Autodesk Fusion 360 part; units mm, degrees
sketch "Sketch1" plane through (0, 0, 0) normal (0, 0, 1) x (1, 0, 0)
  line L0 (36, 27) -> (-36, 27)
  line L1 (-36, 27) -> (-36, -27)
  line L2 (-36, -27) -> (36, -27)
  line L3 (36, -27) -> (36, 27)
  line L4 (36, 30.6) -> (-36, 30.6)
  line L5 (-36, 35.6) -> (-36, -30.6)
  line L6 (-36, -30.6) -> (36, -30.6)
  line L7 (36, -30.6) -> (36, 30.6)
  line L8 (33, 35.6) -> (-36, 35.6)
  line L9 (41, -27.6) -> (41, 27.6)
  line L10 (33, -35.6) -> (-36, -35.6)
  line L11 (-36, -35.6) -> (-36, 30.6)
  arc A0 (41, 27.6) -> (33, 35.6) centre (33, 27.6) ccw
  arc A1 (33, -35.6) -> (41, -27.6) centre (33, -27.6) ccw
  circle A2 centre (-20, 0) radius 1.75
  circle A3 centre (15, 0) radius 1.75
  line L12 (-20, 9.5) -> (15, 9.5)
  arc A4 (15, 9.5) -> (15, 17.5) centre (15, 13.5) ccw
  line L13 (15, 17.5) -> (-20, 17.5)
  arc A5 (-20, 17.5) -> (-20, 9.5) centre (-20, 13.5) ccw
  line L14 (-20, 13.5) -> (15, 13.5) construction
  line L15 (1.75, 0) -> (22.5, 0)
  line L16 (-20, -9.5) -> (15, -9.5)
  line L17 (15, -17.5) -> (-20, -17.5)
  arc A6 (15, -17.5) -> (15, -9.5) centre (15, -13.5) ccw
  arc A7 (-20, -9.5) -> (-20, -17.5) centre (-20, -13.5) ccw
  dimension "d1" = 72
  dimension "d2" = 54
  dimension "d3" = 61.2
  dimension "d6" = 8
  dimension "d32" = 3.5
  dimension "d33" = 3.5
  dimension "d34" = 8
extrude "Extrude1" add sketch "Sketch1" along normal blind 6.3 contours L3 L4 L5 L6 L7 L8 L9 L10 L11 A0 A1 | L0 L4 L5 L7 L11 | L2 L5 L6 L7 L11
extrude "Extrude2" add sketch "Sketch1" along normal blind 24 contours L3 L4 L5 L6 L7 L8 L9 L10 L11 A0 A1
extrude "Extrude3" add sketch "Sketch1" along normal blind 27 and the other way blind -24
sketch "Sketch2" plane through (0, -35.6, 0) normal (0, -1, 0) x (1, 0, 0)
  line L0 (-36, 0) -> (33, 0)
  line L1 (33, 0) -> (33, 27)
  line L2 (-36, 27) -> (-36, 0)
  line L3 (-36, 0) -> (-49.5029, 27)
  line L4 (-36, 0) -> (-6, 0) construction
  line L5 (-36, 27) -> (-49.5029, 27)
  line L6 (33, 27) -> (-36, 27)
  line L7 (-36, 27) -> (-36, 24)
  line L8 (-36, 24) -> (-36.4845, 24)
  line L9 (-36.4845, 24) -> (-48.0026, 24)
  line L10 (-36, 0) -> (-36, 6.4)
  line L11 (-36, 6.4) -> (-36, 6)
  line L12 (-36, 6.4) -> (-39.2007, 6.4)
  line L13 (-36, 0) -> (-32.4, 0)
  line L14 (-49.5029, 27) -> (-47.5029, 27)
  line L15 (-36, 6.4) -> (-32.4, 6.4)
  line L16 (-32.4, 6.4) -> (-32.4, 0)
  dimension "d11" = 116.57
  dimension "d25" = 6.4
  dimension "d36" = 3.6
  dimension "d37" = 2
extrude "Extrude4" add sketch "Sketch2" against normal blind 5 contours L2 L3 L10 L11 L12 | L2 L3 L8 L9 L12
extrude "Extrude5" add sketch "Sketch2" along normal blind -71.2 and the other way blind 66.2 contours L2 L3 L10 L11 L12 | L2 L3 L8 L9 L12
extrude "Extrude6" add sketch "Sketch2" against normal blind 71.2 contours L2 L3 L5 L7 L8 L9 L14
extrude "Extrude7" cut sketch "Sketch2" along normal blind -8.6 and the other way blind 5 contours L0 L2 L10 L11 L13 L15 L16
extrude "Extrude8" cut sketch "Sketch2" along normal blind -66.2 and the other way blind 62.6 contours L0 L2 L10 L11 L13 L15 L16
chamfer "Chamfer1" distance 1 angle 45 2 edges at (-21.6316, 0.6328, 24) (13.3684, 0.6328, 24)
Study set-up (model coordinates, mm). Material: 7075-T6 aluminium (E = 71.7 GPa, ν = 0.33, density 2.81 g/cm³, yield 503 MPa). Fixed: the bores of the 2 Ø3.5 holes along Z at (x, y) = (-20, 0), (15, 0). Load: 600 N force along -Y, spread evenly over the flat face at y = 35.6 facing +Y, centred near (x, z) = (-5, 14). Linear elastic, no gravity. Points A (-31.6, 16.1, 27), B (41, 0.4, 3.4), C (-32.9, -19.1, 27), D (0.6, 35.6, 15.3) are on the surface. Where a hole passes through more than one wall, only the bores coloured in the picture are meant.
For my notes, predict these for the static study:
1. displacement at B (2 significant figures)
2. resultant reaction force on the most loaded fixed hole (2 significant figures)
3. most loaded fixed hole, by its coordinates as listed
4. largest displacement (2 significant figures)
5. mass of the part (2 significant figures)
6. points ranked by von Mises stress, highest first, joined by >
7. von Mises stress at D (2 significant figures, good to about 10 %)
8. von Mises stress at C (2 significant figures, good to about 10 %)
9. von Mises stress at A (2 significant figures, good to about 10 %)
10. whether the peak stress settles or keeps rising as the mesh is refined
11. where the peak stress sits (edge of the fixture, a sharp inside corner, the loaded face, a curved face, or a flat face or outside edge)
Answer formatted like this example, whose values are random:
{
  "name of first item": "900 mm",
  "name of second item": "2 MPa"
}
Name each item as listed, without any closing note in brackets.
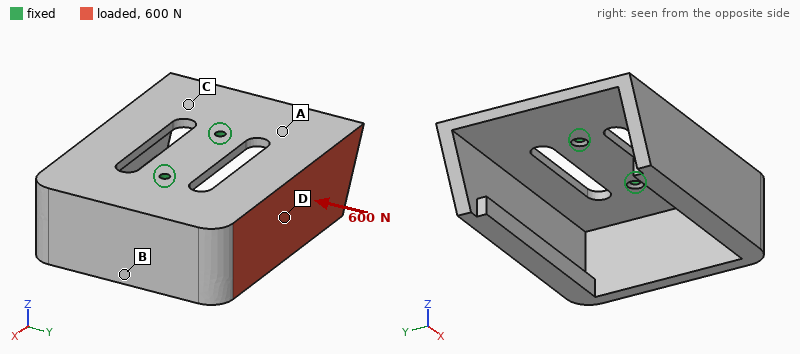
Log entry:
{
  "displacement at B": "0.26 mm",
  "resultant reaction force on the most loaded fixed hole": "350 N",
  "most loaded fixed hole, by its coordinates as listed": "(-20, 0)",
  "largest displacement": "0.55 mm",
  "mass of the part": "130 g",
  "points ranked by von Mises stress, highest first, joined by >": "A > C > D > B",
  "von Mises stress at D": "14 MPa",
  "von Mises stress at C": "29 MPa",
  "von Mises stress at A": "41 MPa",
  "whether the peak stress settles or keeps rising as the mesh is refined": "keeps rising",
  "where the peak stress sits": "edge of the fixture"
}
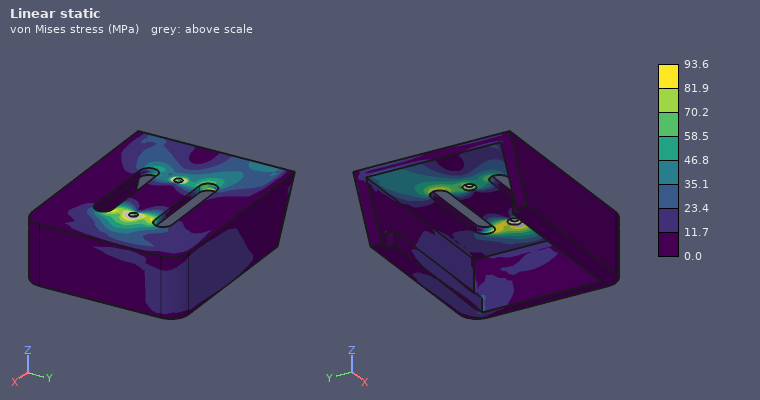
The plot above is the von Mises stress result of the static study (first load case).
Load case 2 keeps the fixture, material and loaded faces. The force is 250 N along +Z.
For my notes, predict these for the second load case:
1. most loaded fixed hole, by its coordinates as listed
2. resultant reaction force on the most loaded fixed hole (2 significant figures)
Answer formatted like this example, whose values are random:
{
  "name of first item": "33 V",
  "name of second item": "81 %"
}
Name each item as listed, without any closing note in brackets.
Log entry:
{
  "most loaded fixed hole, by its coordinates as listed": "(-20, 0)",
  "resultant reaction force on the most loaded fixed hole": "150 N"
}
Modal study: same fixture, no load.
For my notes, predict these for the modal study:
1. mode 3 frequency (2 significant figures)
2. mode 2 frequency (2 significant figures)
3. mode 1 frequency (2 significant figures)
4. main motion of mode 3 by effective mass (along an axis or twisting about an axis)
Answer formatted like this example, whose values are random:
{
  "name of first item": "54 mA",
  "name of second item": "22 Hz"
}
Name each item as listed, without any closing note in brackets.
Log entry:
{
  "mode 3 frequency": "1200 Hz",
  "mode 2 frequency": "950 Hz",
  "mode 1 frequency": "410 Hz",
  "main motion of mode 3 by effective mass": "along Z"
}
